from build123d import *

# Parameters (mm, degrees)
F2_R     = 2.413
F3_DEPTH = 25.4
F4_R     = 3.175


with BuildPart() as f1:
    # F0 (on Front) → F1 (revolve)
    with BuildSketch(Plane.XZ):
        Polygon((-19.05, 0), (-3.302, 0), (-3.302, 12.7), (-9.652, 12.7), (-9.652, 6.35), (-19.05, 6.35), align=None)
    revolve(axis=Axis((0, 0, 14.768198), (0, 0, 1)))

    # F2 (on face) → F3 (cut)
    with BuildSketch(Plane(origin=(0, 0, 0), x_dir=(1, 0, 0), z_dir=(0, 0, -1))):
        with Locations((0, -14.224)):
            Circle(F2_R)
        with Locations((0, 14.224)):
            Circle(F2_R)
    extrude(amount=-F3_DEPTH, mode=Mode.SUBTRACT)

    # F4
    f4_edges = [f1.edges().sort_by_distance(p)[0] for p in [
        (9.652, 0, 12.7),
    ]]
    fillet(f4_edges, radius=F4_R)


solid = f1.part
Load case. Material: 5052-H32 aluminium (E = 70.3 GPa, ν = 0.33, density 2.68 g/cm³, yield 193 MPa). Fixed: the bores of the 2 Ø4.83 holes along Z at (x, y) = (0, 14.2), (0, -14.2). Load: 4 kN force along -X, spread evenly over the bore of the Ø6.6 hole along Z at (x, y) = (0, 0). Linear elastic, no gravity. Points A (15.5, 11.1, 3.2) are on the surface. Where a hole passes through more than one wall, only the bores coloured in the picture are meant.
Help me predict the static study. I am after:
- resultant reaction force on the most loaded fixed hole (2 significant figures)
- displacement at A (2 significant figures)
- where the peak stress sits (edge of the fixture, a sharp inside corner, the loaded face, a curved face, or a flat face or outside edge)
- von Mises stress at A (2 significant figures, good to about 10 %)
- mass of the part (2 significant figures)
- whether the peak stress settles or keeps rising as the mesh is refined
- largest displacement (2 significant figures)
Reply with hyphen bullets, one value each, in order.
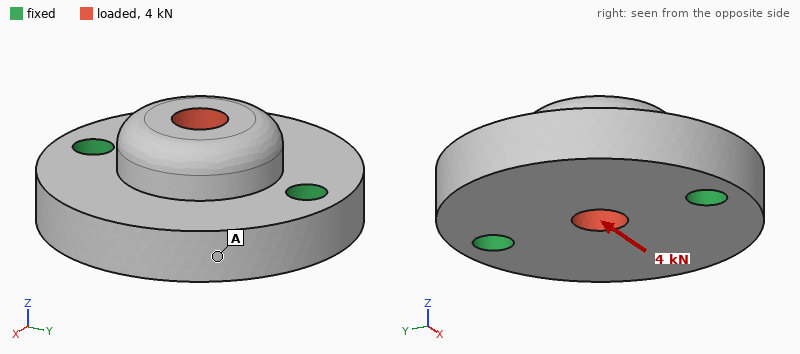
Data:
- 2.0 kN
- 12 µm
- edge of the fixture
- 13 MPa
- 22 g
- keeps rising
- 20 µm
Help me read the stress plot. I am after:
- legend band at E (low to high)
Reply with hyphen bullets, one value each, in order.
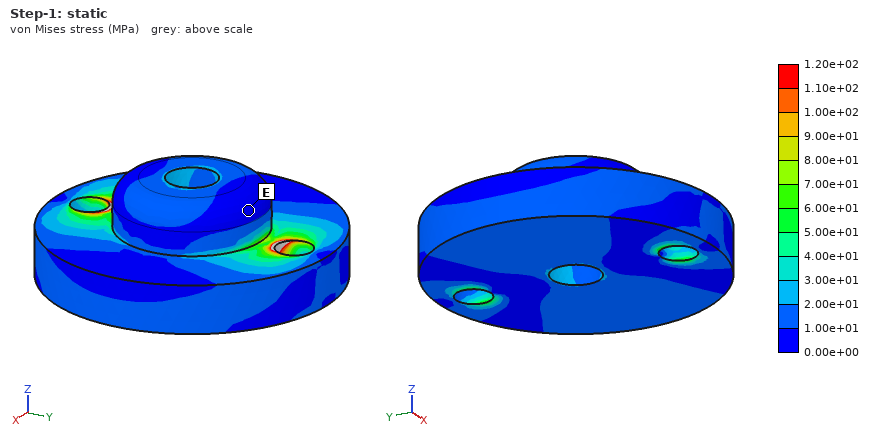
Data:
- 0.00e+00 to 1.00e+01 MPa
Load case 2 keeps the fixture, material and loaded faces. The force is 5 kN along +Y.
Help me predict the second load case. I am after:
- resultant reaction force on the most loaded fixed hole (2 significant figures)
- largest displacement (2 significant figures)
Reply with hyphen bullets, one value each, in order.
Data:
- 2.6 kN
- 8.2 µm
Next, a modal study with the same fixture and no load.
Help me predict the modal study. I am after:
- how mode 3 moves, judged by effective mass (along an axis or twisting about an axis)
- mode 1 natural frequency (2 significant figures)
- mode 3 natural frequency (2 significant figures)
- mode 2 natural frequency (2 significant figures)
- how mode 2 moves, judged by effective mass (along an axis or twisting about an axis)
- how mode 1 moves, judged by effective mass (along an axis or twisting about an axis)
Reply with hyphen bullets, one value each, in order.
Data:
- twisting about X
- 13 kHz
- 36 kHz
- 20 kHz
- along Z
- twisting about Y
